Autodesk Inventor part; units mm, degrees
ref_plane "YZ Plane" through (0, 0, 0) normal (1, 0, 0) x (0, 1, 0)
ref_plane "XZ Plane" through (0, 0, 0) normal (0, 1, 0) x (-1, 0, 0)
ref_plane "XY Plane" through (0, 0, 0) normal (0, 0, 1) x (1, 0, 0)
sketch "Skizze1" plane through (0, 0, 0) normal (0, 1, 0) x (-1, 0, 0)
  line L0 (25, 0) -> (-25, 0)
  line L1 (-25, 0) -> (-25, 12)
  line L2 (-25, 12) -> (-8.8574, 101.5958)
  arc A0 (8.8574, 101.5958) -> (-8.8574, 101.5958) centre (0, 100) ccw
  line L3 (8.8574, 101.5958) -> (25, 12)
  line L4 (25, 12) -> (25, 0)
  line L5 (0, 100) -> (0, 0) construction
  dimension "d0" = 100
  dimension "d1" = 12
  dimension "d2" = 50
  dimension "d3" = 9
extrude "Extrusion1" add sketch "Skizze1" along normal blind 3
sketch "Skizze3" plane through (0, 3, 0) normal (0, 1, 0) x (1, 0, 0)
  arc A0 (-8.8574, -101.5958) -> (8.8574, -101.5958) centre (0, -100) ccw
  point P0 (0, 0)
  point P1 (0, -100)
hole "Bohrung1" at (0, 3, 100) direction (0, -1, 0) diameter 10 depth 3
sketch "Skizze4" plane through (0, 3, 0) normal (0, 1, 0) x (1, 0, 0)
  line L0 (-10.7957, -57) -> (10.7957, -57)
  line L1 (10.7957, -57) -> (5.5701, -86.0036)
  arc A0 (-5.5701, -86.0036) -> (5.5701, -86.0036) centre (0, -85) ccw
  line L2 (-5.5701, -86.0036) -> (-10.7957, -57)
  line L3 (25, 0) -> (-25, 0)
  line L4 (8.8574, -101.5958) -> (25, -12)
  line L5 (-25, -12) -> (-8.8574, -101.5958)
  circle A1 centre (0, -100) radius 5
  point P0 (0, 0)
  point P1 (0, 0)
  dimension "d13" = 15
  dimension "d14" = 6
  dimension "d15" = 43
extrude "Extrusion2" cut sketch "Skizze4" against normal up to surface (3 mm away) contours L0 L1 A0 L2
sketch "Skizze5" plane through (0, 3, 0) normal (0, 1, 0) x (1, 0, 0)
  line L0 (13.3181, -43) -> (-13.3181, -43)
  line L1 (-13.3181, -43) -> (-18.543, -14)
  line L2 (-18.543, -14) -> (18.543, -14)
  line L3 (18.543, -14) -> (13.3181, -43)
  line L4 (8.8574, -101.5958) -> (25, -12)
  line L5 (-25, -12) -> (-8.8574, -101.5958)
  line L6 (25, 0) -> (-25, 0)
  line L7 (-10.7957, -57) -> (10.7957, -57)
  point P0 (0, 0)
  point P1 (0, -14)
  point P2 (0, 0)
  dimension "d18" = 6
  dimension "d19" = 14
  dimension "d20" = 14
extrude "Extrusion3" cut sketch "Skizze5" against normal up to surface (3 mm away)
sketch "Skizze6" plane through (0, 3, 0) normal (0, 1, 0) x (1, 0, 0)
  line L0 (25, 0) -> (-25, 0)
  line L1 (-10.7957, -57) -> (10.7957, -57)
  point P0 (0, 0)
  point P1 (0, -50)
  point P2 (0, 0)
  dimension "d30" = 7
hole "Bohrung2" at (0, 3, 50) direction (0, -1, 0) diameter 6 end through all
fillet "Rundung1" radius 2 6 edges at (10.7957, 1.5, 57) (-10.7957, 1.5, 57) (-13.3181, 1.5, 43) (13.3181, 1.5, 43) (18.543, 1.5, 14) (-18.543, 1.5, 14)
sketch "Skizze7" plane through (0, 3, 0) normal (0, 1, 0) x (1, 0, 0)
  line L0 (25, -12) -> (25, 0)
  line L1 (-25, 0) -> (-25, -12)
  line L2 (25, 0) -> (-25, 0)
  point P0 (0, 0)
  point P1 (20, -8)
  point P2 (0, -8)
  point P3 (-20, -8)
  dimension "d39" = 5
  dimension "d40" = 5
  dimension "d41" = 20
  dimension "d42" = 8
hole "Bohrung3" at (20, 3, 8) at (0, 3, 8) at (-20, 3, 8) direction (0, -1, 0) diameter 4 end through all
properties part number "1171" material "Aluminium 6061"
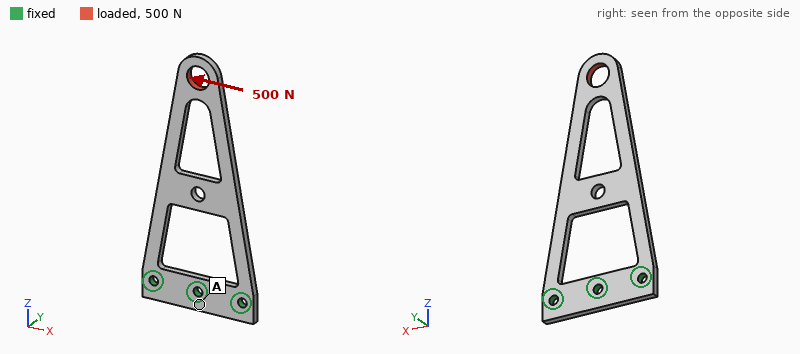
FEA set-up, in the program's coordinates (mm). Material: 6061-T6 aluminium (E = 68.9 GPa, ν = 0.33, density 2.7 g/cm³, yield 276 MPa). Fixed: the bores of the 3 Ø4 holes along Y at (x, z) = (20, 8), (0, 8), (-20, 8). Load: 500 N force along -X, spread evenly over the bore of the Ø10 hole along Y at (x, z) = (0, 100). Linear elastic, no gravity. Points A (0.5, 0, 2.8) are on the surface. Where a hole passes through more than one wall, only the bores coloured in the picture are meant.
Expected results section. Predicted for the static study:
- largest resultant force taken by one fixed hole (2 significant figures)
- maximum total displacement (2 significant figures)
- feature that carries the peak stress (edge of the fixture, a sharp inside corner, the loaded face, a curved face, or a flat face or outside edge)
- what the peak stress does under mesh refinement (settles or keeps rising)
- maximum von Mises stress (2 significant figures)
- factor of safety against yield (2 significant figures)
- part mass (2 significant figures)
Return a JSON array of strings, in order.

["1.1 kN", "0.34 mm", "a curved face", "settles", "180 MPa", "1.5", "17 g"]
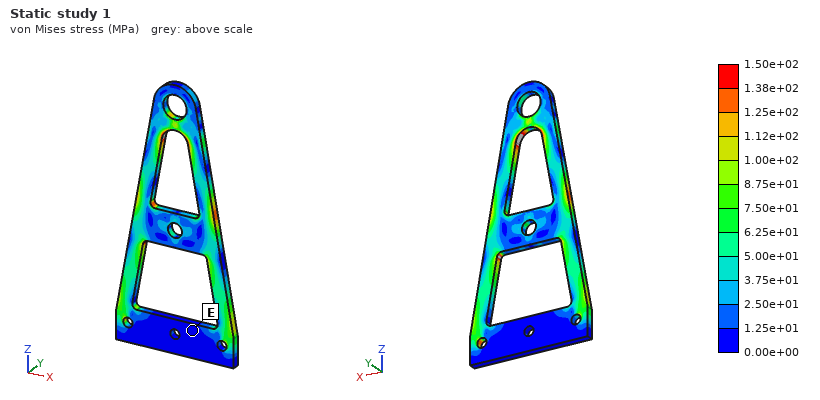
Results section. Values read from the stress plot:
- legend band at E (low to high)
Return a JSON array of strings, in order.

["0.00e+00 to 1.25e+01 MPa"]
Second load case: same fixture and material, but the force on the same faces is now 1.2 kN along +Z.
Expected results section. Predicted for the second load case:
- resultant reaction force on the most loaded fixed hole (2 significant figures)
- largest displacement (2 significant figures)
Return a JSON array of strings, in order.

["630 N", "49 µm"]
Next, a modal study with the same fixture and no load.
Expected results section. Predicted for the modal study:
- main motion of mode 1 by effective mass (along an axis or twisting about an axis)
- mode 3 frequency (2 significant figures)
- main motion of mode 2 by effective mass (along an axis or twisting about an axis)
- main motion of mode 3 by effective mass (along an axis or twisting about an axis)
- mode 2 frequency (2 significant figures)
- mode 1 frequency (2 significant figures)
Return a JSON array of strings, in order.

["along Y", "1600 Hz", "along Y", "twisting about Z", "1400 Hz", "250 Hz"]
